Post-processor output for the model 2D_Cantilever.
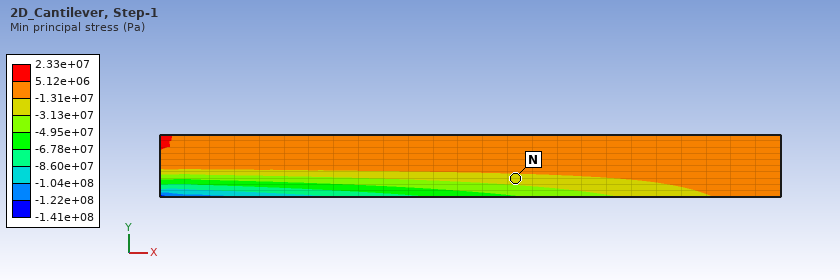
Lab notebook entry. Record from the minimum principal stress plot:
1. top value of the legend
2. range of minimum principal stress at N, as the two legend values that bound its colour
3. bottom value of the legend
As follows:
2.33e+07 Pa
-3.13e+07 to -1.31e+07 Pa
-1.41e+08 Pa
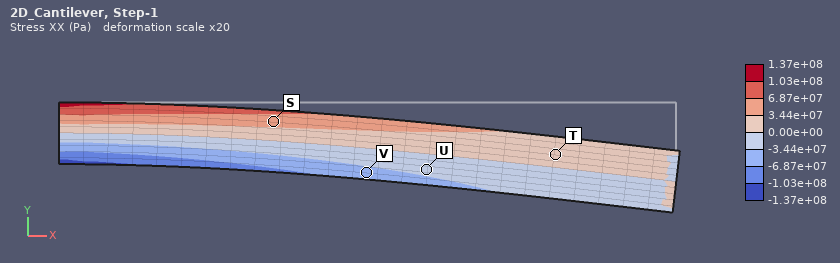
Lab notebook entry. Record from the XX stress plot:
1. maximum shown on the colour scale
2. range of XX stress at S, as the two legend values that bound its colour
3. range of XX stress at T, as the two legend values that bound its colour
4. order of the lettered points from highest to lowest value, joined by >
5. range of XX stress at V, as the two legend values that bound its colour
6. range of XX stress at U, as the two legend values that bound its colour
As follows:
1.37e+08 Pa
3.44e+07 to 6.87e+07 Pa
0.00e+00 to 3.44e+07 Pa
S > T > U > V
-6.87e+07 to -3.44e+07 Pa
-3.44e+07 to 0.00e+00 Pa
